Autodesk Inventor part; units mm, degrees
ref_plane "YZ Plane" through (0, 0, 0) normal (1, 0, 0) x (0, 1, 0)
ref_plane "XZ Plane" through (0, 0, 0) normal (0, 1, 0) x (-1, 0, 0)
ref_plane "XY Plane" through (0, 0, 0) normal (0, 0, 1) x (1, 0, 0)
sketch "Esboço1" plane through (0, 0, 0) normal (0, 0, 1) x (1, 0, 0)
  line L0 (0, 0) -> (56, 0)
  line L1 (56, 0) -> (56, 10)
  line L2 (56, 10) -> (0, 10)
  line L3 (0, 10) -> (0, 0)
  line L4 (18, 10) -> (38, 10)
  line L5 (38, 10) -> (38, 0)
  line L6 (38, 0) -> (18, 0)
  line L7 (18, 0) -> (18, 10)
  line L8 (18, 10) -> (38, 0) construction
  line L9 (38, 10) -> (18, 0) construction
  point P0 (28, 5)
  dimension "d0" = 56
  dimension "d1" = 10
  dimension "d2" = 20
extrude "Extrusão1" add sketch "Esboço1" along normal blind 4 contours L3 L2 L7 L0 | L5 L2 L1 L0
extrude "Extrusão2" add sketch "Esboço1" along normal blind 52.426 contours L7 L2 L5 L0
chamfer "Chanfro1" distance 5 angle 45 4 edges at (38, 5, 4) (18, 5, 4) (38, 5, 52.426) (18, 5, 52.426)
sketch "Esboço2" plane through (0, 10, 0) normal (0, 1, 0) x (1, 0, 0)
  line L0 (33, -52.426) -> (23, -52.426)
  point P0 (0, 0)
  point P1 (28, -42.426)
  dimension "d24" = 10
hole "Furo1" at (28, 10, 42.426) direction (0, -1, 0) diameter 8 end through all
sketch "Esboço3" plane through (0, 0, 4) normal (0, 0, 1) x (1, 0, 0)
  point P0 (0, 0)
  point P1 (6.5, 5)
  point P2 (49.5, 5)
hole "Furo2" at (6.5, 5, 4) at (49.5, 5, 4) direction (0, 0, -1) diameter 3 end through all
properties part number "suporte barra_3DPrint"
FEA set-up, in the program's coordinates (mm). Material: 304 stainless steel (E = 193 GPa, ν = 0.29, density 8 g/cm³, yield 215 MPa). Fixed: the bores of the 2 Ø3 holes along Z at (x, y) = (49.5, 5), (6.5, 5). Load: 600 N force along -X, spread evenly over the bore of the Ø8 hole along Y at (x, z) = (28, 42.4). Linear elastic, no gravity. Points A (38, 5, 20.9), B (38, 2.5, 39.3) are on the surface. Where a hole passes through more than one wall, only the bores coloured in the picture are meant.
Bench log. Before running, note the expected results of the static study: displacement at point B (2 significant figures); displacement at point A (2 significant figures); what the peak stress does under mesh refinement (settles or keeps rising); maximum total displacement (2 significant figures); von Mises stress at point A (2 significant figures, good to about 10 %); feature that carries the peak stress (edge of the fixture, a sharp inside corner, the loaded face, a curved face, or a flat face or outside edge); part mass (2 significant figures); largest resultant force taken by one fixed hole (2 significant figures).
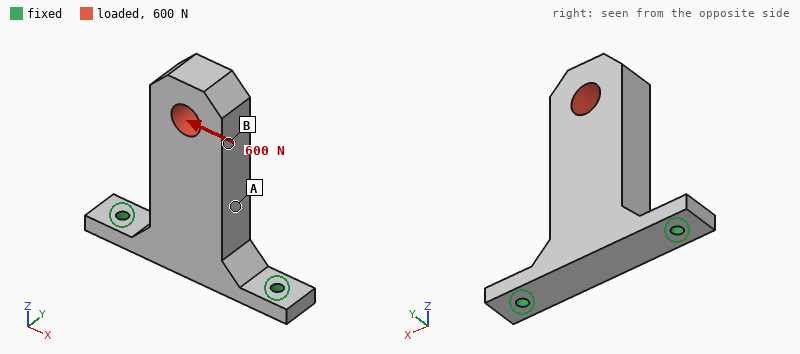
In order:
26 µm
12 µm
keeps rising
35 µm
19 MPa
edge of the fixture
91 g
760 N
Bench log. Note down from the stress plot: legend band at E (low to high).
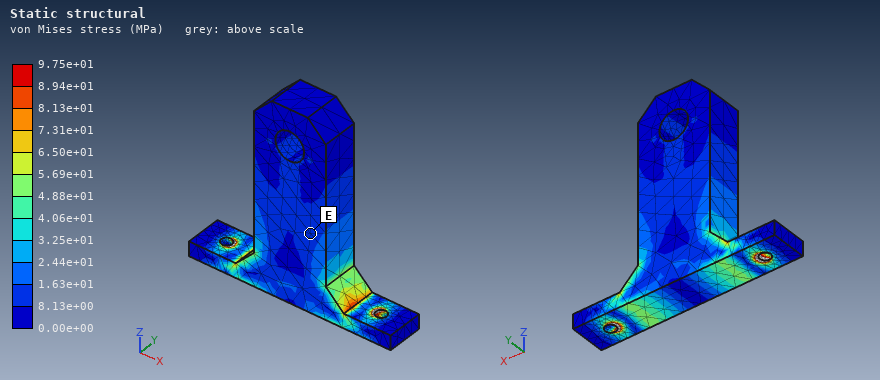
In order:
8.13e+00 to 1.63e+01 MPa
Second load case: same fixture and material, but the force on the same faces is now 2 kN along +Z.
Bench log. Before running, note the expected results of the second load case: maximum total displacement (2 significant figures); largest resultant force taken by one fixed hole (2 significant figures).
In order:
14 µm
1.3 kN
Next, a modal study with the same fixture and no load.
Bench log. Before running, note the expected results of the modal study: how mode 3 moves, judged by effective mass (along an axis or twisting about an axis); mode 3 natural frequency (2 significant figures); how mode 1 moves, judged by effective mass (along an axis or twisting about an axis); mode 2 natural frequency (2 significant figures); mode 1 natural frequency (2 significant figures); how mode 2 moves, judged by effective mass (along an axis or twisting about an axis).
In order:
along Z
7200 Hz
along Y
4000 Hz
1100 Hz
along X
